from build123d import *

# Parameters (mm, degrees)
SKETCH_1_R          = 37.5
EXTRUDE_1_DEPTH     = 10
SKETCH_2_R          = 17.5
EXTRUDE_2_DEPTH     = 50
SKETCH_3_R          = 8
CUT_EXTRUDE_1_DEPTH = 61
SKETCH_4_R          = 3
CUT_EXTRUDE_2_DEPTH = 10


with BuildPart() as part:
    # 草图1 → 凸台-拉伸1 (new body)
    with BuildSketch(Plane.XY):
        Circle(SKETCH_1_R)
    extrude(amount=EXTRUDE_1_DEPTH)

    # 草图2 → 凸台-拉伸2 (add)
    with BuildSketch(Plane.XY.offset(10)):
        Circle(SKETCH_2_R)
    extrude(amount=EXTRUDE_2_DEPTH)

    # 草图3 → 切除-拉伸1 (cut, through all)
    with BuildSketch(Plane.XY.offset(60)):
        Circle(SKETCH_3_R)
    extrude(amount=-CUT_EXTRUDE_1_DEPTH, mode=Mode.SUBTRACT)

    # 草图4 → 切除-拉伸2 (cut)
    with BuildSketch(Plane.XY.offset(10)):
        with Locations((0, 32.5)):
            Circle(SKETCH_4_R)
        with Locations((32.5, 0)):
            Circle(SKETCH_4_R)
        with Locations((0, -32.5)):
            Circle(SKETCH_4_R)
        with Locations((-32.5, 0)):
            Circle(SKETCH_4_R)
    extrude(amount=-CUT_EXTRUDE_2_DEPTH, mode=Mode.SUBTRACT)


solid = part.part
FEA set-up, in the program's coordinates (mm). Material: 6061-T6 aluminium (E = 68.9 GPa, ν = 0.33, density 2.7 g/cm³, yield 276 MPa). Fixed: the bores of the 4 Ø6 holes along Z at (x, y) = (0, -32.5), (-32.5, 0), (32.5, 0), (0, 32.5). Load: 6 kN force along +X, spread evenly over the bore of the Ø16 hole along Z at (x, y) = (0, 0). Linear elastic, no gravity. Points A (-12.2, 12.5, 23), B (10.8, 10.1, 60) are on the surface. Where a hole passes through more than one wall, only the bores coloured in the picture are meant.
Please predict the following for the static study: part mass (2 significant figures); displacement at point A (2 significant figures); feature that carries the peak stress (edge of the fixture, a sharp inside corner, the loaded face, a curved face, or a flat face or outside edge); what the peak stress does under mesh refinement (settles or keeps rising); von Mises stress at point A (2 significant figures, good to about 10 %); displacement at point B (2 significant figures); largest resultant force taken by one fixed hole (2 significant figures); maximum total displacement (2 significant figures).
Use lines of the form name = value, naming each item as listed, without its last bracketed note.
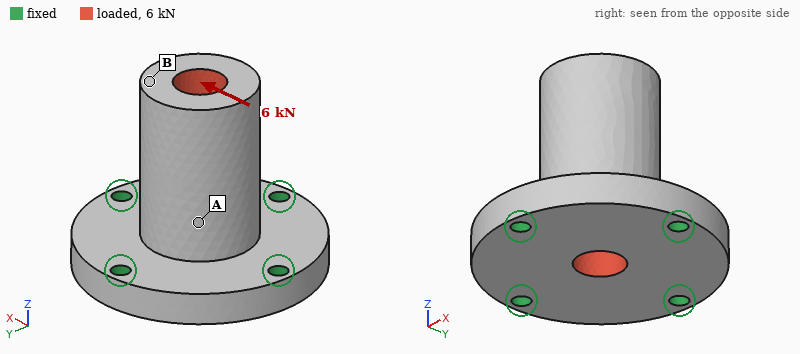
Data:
part mass = 210 g
displacement at point A = 24 µm
feature that carries the peak stress = edge of the fixture
what the peak stress does under mesh refinement = keeps rising
von Mises stress at point A = 13 MPa
displacement at point B = 70 µm
largest resultant force taken by one fixed hole = 3.3 kN
maximum total displacement = 72 µm
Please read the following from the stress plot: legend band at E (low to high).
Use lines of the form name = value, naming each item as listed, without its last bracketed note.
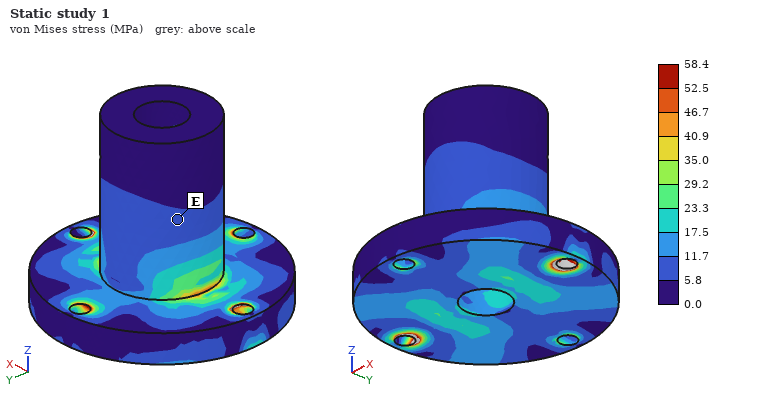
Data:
legend band at E = 5.8 to 11.7 MPa
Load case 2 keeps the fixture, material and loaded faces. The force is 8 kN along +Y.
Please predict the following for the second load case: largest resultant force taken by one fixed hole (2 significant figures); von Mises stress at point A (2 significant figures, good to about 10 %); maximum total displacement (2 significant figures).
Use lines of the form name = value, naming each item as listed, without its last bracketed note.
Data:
largest resultant force taken by one fixed hole = 4.3 kN
von Mises stress at point A = 18 MPa
maximum total displacement = 97 µm
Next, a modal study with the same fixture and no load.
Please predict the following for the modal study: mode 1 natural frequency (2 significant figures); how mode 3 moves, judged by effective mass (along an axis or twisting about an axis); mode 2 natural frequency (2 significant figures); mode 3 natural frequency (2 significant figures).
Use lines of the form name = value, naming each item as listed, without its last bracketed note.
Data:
mode 1 natural frequency = 4900 Hz
how mode 3 moves, judged by effective mass = along Z
mode 2 natural frequency = 4900 Hz
mode 3 natural frequency = 9300 Hz
